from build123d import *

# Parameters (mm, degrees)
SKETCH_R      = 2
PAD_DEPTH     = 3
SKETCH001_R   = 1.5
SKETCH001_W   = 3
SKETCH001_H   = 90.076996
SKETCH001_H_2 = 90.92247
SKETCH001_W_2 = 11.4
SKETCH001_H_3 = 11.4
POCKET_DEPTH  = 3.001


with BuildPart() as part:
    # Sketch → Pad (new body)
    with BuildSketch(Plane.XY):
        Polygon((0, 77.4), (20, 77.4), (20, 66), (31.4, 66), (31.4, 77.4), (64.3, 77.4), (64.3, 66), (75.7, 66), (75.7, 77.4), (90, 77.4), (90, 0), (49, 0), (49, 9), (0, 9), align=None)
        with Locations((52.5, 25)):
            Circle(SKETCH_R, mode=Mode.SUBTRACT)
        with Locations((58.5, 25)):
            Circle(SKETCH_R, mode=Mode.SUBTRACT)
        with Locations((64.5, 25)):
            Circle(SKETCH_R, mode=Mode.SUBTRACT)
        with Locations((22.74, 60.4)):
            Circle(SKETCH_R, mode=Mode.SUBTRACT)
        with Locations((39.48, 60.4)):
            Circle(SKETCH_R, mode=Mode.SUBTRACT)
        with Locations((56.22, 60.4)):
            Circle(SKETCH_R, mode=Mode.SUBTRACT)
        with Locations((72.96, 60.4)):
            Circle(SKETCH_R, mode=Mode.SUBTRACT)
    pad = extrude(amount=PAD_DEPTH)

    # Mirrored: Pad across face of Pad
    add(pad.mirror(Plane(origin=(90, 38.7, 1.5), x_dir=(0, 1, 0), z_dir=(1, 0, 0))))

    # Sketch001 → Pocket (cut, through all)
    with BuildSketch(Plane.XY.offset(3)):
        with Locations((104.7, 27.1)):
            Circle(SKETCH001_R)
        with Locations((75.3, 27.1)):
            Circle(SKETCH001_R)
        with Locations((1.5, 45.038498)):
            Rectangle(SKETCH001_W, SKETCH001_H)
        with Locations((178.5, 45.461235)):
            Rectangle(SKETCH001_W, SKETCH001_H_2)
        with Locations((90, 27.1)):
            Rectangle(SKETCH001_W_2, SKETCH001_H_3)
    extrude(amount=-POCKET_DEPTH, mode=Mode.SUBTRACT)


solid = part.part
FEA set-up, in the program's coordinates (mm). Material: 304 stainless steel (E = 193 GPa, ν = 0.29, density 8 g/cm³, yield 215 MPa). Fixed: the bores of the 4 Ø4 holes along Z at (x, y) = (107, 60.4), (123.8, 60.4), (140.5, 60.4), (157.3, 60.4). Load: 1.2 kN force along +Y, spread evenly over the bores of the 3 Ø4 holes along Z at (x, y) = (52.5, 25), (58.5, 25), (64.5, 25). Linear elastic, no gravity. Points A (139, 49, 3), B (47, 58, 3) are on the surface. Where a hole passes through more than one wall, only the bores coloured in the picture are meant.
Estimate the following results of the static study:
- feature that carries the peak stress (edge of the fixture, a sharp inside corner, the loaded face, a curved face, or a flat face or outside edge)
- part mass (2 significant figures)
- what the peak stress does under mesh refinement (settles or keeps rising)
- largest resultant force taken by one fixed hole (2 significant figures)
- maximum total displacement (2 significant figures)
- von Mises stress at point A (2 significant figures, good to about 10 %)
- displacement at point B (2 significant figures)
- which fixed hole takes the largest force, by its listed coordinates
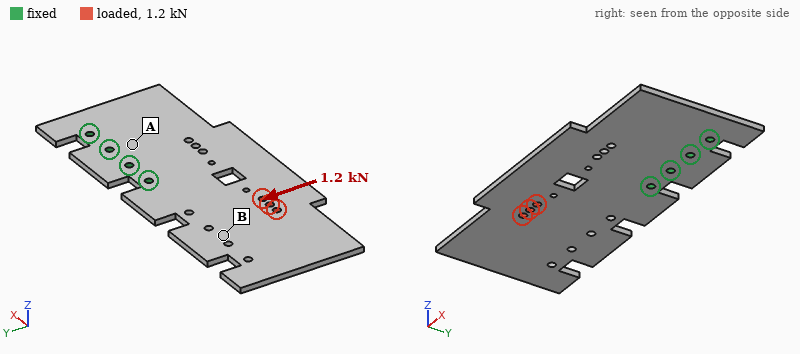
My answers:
edge of the fixture
280 g
keeps rising
2.2 kN
44 µm
17 MPa
27 µm
(107, 60.4)
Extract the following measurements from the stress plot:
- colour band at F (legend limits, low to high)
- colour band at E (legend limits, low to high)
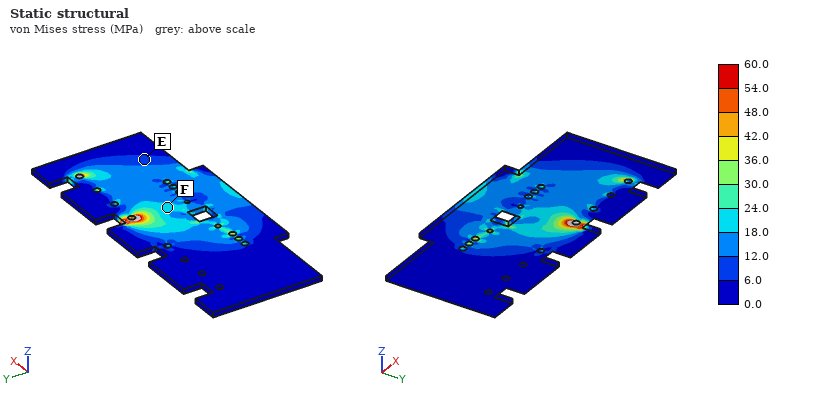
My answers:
18.0 to 24.0 MPa
6.0 to 12.0 MPa
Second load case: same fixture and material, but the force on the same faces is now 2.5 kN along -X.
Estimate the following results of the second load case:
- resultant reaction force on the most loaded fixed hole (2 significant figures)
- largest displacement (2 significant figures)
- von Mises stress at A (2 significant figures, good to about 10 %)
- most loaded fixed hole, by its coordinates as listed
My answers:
1.8 kN
46 µm
26 MPa
(107, 60.4)
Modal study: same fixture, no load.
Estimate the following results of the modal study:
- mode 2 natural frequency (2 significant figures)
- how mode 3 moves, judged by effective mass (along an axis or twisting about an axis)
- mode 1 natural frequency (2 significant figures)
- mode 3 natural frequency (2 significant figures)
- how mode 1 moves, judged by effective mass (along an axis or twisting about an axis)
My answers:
480 Hz
along Z
190 Hz
930 Hz
along Z
